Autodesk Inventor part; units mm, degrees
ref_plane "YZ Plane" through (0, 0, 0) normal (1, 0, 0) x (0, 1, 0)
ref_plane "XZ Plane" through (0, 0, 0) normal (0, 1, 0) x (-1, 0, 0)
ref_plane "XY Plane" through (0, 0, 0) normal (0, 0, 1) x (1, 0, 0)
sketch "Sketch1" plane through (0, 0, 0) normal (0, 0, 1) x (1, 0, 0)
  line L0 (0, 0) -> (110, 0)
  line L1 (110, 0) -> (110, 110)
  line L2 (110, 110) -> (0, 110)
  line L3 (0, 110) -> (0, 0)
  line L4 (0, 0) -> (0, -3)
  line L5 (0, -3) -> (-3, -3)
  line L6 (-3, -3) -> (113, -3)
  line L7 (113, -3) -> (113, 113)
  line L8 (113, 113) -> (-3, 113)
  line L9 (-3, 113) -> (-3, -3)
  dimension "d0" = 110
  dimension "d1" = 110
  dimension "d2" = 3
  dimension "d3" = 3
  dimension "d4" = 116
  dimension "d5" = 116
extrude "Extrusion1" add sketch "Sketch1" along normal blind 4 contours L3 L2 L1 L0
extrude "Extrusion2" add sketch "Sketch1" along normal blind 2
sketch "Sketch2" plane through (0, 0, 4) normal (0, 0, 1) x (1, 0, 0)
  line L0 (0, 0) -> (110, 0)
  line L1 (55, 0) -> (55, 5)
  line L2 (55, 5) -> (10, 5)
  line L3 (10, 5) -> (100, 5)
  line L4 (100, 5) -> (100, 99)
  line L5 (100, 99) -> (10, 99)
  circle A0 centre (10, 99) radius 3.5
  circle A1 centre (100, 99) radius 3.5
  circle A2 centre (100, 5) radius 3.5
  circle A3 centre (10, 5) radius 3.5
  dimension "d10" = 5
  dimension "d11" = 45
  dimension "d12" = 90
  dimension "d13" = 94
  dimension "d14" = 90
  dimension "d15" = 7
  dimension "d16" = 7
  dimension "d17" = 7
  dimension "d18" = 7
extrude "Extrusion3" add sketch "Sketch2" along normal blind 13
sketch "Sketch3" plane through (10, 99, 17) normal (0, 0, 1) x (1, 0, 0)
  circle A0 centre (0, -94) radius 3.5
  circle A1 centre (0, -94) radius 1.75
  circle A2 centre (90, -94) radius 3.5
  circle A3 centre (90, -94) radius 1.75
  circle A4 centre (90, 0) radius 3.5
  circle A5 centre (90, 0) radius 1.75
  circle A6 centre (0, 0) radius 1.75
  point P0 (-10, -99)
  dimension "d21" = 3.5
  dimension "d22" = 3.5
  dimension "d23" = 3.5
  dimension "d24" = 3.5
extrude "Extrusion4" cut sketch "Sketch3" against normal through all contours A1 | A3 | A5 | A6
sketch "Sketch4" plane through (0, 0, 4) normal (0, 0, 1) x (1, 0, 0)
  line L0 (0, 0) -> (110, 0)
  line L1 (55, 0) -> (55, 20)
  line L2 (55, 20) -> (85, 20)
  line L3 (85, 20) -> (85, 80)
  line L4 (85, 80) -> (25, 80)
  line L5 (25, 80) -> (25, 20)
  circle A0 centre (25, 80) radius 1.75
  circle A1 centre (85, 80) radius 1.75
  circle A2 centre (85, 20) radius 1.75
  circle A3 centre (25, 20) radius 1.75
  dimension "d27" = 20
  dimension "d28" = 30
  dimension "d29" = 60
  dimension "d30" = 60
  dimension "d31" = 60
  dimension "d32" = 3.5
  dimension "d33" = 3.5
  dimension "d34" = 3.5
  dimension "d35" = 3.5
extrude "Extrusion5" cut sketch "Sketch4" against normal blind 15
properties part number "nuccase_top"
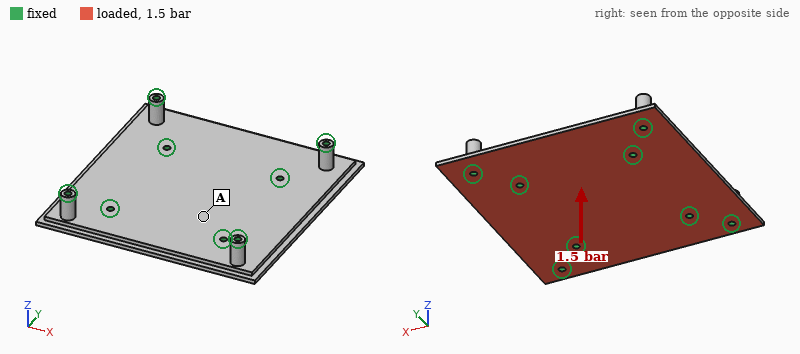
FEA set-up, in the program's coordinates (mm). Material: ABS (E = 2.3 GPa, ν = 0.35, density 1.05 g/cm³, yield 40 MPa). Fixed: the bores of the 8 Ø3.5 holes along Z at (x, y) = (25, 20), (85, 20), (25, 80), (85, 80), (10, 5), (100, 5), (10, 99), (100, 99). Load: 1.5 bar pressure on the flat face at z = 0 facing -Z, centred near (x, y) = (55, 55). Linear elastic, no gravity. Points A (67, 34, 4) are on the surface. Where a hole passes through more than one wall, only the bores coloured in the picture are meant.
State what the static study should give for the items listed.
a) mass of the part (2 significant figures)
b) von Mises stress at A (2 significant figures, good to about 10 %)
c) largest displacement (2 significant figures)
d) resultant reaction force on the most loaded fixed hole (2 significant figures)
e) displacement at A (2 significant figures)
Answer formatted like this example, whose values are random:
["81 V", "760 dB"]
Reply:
["55 g", "5.5 MPa", "1.4 mm", "400 N", "0.62 mm"]
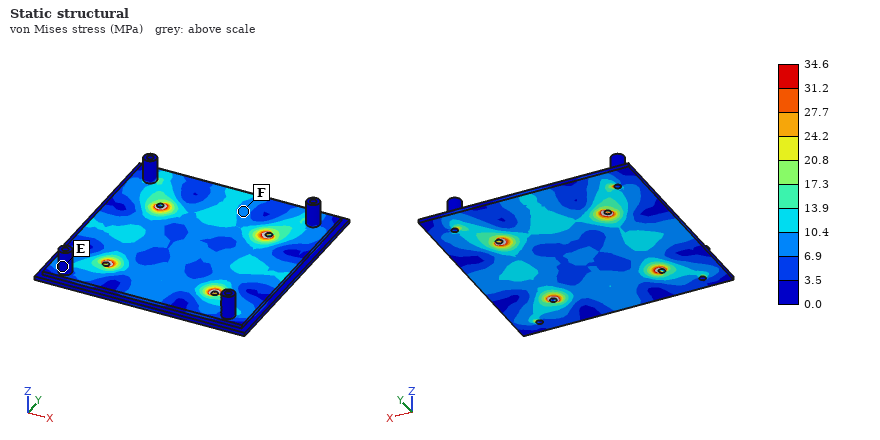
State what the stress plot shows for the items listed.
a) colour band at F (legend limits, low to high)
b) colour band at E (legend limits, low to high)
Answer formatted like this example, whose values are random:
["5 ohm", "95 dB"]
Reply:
["6.9 to 10.4 MPa", "0.0 to 3.5 MPa"]
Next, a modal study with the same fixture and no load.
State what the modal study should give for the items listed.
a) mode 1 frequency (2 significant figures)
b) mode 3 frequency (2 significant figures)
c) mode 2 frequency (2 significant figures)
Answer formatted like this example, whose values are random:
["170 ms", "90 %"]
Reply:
["1000 Hz", "1200 Hz", "1100 Hz"]
